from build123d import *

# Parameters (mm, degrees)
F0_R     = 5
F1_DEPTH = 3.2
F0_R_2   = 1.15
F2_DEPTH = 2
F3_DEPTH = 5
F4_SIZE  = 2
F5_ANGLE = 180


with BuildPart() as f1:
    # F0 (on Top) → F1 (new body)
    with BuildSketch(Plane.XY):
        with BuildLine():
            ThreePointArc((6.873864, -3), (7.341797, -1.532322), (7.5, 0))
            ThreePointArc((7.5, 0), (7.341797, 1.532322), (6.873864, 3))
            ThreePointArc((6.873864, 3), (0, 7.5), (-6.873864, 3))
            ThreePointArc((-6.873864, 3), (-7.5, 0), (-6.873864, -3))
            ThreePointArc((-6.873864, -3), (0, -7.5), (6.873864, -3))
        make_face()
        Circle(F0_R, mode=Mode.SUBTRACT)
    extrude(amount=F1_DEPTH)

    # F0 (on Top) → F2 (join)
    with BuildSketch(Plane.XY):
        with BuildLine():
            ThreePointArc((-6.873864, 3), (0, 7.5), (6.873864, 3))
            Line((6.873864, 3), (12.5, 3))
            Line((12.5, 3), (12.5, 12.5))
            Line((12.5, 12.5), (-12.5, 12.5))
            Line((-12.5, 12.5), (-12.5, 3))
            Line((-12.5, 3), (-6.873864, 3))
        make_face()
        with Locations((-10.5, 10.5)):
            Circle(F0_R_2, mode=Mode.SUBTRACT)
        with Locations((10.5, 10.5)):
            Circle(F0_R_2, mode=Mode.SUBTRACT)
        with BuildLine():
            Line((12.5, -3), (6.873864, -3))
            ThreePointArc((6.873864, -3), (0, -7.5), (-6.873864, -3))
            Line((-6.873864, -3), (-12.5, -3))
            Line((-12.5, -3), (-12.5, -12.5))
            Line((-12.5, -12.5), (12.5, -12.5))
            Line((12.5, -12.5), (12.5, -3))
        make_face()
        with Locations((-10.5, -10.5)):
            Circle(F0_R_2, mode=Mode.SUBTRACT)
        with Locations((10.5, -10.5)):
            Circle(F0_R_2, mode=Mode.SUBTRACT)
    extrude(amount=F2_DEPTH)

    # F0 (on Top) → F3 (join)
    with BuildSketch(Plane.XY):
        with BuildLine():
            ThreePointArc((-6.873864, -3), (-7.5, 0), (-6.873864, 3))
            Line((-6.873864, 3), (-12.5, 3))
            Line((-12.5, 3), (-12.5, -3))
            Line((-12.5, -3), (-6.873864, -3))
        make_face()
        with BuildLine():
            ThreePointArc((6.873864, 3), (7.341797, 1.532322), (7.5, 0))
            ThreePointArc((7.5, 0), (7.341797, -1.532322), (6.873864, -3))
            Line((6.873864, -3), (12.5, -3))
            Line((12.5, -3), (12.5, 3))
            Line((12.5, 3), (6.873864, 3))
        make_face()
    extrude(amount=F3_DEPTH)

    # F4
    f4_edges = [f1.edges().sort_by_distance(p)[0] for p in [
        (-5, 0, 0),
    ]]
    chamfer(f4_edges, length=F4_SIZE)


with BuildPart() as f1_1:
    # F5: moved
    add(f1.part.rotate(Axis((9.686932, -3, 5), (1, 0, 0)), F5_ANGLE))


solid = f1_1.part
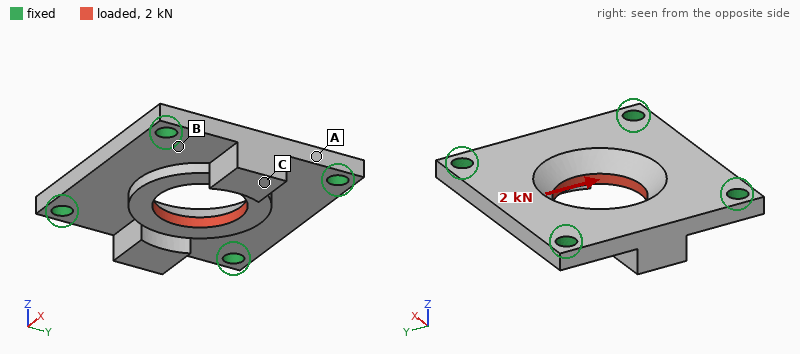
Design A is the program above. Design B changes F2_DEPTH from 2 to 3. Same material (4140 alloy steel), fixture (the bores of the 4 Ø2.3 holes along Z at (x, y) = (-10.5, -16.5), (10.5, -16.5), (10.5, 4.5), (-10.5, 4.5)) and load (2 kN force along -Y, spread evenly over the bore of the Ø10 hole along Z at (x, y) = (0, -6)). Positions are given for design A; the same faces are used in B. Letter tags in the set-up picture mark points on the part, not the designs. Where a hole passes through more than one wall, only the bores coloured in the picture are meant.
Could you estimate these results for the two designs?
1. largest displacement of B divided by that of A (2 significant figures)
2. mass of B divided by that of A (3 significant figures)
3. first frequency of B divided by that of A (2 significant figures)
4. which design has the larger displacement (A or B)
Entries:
0.61
1.29
1.3
A
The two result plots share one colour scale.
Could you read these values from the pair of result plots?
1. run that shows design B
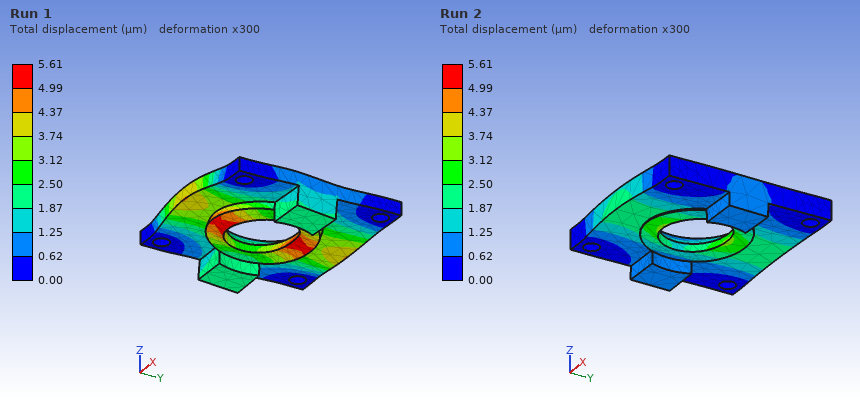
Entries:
Run 2
